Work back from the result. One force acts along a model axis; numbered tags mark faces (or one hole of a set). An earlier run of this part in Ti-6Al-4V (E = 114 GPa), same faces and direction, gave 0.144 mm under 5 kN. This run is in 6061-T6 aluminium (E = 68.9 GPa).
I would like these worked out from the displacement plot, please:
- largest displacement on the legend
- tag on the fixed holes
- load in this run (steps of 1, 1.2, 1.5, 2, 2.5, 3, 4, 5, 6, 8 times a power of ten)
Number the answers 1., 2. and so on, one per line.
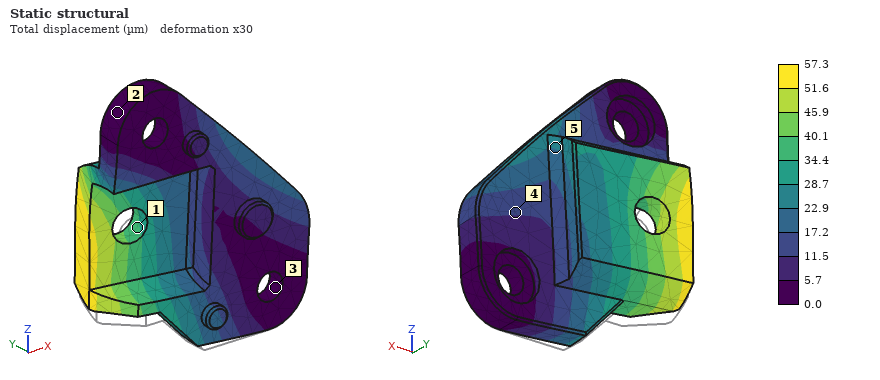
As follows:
1. 57.3 µm
2. 3
3. 1.2 kN
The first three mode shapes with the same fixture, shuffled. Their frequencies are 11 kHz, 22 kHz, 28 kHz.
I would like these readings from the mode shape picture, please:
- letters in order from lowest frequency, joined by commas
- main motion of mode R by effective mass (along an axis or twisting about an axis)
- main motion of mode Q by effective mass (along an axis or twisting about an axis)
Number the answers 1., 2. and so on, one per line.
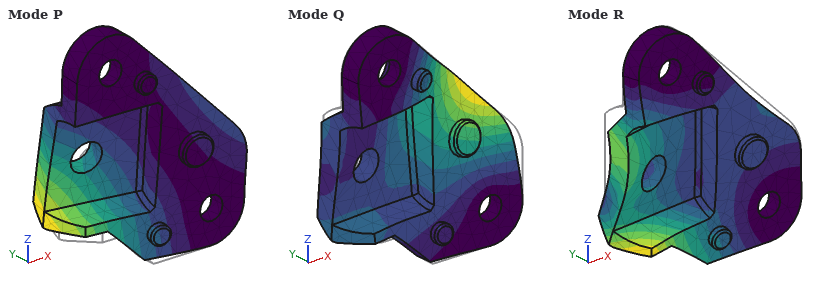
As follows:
1. P, Q, R
2. along Z
3. along Y
